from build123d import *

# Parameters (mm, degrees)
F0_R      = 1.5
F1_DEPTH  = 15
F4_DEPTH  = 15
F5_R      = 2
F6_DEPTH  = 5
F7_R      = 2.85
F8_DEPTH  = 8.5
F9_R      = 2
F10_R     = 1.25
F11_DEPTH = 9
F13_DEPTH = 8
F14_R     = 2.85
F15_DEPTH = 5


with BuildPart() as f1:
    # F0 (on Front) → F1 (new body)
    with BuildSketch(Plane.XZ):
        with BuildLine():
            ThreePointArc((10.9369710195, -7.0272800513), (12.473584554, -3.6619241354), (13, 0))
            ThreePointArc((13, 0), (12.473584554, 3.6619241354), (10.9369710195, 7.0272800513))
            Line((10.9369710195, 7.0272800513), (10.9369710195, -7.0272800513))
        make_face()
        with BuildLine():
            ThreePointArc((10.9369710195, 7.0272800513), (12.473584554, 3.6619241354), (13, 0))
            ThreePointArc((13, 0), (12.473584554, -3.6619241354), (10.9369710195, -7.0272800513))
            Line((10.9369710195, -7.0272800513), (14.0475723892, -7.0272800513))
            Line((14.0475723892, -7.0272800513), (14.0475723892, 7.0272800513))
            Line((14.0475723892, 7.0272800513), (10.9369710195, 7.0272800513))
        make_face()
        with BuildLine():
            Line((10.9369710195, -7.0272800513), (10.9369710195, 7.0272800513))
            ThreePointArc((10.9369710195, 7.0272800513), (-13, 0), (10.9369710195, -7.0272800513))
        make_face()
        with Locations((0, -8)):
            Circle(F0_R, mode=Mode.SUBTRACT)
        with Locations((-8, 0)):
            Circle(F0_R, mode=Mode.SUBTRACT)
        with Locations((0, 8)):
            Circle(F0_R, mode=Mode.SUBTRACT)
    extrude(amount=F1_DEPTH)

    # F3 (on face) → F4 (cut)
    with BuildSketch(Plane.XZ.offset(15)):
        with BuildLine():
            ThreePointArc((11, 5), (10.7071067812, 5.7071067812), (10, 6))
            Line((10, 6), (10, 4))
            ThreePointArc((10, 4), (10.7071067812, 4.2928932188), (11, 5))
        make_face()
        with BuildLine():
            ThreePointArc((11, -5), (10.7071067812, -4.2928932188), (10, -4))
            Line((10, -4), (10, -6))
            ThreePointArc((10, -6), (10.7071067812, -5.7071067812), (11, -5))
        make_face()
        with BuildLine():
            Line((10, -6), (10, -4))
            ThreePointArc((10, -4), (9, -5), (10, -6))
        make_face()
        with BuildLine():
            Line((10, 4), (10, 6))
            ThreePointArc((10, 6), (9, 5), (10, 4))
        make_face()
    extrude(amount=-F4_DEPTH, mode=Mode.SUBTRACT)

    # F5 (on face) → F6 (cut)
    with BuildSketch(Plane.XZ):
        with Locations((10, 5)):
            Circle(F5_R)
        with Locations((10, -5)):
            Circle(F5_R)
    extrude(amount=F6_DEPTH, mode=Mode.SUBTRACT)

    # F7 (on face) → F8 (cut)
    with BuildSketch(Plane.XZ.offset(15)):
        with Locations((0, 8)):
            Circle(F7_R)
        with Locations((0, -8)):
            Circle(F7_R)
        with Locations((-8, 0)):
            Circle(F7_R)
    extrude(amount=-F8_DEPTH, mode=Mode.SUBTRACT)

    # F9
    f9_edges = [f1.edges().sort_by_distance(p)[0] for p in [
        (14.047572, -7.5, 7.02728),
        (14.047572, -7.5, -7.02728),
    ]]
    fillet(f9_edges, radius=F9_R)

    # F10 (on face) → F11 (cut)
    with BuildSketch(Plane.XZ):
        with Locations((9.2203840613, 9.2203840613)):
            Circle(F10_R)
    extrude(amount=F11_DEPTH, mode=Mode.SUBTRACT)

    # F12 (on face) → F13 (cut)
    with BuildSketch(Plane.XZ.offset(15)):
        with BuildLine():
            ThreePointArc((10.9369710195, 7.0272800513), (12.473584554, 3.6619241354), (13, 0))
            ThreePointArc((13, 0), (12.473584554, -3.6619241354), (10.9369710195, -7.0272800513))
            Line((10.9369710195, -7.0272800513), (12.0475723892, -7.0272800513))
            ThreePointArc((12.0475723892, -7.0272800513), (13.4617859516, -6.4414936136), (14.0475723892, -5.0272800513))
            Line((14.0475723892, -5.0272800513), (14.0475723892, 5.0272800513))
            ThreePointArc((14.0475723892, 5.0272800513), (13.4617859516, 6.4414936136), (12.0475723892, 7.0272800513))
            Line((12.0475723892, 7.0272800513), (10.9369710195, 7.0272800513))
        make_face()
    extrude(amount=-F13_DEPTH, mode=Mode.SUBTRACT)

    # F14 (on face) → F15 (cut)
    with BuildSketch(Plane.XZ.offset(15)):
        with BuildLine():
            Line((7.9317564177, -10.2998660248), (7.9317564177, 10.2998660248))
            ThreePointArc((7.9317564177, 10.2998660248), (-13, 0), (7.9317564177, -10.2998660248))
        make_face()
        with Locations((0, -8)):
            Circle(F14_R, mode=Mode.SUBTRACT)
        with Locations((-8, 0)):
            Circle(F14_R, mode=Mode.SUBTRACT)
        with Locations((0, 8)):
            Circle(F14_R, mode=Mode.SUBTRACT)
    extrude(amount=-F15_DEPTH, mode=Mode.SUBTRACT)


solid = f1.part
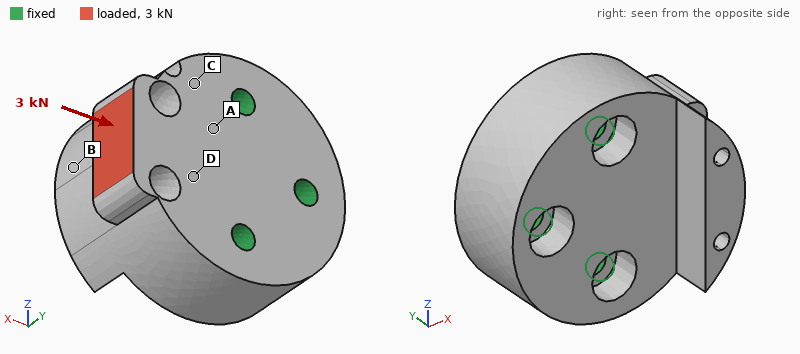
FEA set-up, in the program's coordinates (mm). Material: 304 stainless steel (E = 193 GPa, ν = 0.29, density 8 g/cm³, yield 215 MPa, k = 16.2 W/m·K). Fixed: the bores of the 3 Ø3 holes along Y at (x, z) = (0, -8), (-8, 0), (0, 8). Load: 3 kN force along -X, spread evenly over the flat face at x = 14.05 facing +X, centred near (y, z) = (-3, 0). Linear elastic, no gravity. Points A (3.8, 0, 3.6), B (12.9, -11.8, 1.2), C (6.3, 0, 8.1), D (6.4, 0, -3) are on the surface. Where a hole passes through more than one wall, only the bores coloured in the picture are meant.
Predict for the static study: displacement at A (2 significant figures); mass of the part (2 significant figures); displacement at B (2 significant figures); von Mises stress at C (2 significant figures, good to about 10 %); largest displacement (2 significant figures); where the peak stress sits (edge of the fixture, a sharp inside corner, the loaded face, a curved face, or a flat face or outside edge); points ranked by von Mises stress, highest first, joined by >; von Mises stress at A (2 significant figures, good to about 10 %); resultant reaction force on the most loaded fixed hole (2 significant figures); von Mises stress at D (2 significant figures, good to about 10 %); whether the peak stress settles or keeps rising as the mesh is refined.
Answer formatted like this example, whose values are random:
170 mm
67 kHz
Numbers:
0.90 µm
42 g
1.0 µm
21 MPa
4.5 µm
a sharp inside corner
D > A > C > B
35 MPa
1.2 kN
51 MPa
keeps rising
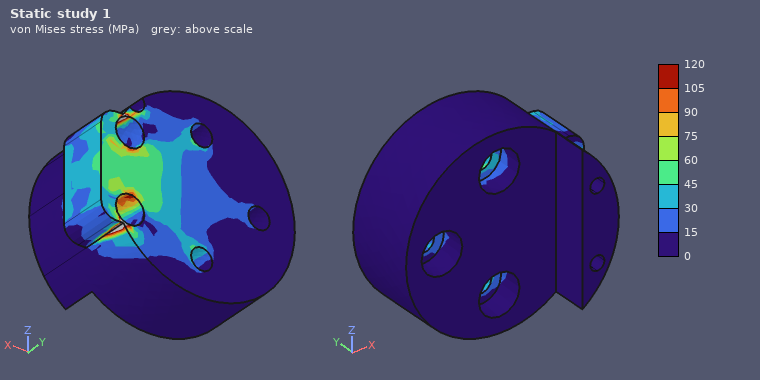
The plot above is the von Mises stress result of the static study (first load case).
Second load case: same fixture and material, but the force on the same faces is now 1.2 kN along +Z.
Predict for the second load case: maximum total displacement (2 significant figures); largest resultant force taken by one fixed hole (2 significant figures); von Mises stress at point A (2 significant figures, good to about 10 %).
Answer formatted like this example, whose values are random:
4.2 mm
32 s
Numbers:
3.9 µm
1.1 kN
19 MPa
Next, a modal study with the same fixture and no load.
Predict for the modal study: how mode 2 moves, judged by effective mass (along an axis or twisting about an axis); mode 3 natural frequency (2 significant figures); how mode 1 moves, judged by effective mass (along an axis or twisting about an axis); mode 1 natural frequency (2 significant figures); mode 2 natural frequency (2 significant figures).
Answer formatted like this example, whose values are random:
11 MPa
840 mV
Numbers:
along Z
47 kHz
along Y
22 kHz
41 kHz
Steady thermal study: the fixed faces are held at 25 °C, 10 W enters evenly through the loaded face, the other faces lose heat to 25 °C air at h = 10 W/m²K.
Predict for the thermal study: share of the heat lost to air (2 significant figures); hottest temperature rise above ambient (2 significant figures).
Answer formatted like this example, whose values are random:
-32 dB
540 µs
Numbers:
4.3 %
82 K
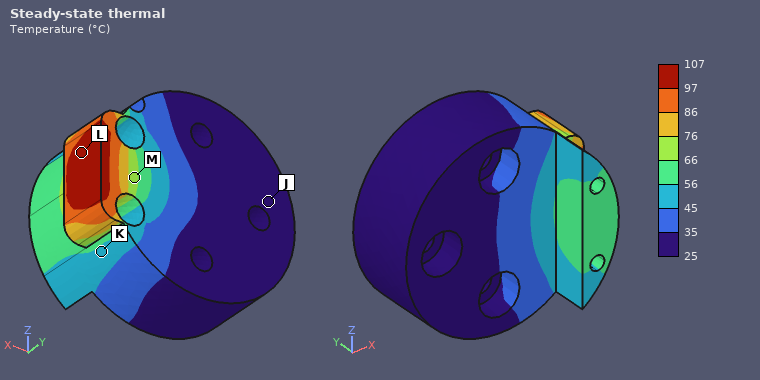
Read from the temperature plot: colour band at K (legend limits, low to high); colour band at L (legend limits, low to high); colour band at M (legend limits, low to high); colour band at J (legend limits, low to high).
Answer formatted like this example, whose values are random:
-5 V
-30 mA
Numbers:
45 to 56 °C
97 to 107 °C
66 to 76 °C
25 to 35 °C
